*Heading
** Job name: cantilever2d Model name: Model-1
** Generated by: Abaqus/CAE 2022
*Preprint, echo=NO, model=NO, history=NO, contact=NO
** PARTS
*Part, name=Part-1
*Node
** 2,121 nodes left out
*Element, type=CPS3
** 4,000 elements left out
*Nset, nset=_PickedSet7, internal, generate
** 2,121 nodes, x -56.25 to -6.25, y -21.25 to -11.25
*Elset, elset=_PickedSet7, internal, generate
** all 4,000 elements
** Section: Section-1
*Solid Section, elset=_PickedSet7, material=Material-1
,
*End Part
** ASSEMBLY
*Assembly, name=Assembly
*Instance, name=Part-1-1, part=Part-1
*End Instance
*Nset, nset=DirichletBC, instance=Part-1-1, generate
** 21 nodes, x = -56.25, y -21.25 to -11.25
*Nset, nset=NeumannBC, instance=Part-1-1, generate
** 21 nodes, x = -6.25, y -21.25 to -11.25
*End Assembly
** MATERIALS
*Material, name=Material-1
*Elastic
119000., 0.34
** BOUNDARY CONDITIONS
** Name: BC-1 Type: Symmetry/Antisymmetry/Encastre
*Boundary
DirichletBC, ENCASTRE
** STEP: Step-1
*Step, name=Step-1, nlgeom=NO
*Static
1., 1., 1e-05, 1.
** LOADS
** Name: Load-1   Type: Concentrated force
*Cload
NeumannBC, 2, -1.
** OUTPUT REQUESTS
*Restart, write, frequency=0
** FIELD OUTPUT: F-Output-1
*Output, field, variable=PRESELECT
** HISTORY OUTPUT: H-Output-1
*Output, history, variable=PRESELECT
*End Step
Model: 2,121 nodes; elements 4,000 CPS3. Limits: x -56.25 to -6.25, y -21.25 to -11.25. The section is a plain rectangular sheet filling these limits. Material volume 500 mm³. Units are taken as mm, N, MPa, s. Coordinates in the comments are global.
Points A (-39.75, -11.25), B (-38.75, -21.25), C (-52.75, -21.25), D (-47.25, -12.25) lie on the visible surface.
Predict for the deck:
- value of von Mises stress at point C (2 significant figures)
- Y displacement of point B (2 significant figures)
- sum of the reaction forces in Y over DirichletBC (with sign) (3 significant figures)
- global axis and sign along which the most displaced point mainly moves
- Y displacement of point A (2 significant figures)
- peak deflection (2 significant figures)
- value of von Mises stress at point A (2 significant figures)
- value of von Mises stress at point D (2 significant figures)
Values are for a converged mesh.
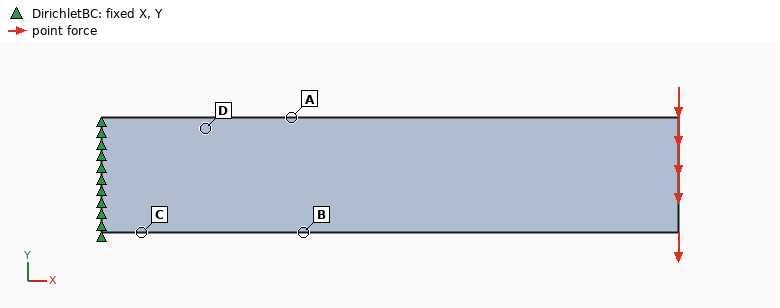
57 MPa
-0.015 mm
21.0 N
-Y
-0.014 mm
0.092 mm
42 MPa
41 MPa
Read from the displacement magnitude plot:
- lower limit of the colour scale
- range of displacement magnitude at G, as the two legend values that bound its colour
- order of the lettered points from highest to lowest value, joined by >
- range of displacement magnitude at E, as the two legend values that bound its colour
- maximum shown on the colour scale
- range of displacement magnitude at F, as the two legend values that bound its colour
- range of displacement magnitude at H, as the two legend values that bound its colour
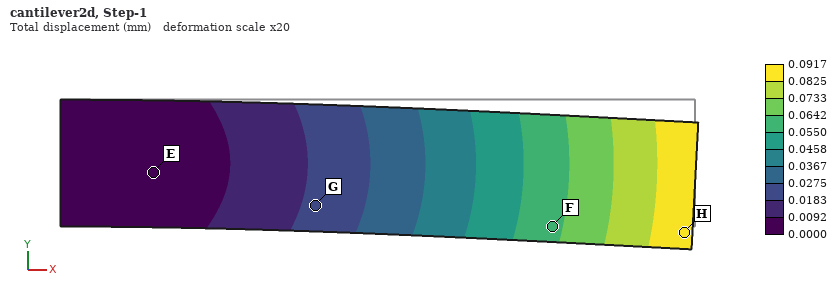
0.0000 mm
0.0183 to 0.0275 mm
H > F > G > E
0.0000 to 0.0092 mm
0.0917 mm
0.0550 to 0.0642 mm
0.0825 to 0.0917 mm
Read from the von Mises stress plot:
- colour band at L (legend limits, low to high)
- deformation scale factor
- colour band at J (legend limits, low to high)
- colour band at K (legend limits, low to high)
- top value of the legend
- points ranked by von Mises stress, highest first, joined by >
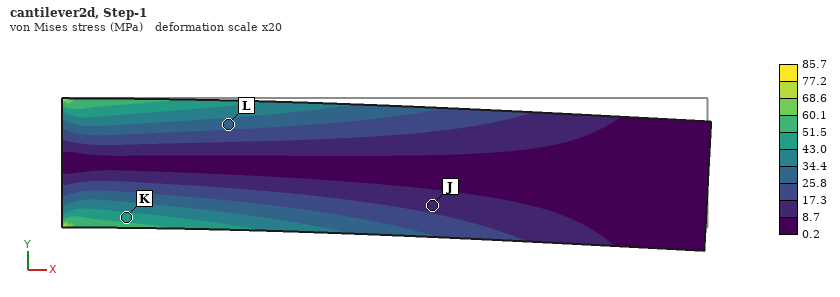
25.8 to 34.4 MPa
20
8.7 to 17.3 MPa
43.0 to 51.5 MPa
85.7 MPa
K > L > J
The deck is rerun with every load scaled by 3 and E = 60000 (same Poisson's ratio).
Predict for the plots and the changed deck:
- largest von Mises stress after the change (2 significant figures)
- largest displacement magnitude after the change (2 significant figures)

260 MPa
0.55 mm
